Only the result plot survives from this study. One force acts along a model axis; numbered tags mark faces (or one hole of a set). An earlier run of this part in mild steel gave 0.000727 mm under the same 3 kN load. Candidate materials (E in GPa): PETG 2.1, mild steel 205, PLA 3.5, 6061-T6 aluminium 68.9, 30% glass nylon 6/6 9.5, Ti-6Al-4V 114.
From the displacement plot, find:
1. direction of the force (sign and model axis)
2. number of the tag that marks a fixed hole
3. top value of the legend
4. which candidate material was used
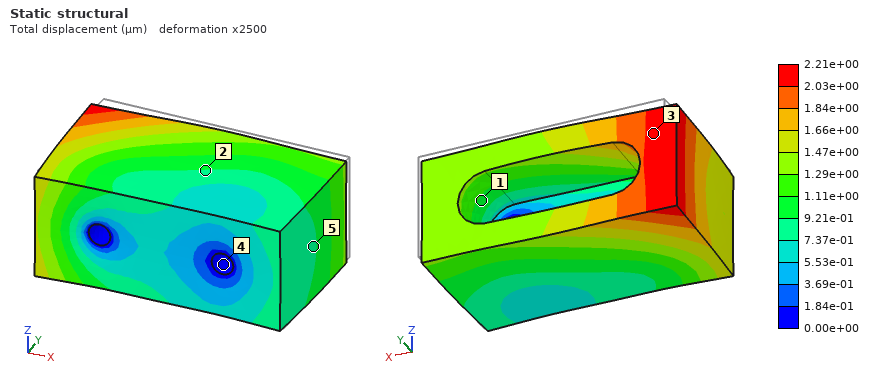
-Y
4
2.21e+00 µm
6061-T6 aluminium
